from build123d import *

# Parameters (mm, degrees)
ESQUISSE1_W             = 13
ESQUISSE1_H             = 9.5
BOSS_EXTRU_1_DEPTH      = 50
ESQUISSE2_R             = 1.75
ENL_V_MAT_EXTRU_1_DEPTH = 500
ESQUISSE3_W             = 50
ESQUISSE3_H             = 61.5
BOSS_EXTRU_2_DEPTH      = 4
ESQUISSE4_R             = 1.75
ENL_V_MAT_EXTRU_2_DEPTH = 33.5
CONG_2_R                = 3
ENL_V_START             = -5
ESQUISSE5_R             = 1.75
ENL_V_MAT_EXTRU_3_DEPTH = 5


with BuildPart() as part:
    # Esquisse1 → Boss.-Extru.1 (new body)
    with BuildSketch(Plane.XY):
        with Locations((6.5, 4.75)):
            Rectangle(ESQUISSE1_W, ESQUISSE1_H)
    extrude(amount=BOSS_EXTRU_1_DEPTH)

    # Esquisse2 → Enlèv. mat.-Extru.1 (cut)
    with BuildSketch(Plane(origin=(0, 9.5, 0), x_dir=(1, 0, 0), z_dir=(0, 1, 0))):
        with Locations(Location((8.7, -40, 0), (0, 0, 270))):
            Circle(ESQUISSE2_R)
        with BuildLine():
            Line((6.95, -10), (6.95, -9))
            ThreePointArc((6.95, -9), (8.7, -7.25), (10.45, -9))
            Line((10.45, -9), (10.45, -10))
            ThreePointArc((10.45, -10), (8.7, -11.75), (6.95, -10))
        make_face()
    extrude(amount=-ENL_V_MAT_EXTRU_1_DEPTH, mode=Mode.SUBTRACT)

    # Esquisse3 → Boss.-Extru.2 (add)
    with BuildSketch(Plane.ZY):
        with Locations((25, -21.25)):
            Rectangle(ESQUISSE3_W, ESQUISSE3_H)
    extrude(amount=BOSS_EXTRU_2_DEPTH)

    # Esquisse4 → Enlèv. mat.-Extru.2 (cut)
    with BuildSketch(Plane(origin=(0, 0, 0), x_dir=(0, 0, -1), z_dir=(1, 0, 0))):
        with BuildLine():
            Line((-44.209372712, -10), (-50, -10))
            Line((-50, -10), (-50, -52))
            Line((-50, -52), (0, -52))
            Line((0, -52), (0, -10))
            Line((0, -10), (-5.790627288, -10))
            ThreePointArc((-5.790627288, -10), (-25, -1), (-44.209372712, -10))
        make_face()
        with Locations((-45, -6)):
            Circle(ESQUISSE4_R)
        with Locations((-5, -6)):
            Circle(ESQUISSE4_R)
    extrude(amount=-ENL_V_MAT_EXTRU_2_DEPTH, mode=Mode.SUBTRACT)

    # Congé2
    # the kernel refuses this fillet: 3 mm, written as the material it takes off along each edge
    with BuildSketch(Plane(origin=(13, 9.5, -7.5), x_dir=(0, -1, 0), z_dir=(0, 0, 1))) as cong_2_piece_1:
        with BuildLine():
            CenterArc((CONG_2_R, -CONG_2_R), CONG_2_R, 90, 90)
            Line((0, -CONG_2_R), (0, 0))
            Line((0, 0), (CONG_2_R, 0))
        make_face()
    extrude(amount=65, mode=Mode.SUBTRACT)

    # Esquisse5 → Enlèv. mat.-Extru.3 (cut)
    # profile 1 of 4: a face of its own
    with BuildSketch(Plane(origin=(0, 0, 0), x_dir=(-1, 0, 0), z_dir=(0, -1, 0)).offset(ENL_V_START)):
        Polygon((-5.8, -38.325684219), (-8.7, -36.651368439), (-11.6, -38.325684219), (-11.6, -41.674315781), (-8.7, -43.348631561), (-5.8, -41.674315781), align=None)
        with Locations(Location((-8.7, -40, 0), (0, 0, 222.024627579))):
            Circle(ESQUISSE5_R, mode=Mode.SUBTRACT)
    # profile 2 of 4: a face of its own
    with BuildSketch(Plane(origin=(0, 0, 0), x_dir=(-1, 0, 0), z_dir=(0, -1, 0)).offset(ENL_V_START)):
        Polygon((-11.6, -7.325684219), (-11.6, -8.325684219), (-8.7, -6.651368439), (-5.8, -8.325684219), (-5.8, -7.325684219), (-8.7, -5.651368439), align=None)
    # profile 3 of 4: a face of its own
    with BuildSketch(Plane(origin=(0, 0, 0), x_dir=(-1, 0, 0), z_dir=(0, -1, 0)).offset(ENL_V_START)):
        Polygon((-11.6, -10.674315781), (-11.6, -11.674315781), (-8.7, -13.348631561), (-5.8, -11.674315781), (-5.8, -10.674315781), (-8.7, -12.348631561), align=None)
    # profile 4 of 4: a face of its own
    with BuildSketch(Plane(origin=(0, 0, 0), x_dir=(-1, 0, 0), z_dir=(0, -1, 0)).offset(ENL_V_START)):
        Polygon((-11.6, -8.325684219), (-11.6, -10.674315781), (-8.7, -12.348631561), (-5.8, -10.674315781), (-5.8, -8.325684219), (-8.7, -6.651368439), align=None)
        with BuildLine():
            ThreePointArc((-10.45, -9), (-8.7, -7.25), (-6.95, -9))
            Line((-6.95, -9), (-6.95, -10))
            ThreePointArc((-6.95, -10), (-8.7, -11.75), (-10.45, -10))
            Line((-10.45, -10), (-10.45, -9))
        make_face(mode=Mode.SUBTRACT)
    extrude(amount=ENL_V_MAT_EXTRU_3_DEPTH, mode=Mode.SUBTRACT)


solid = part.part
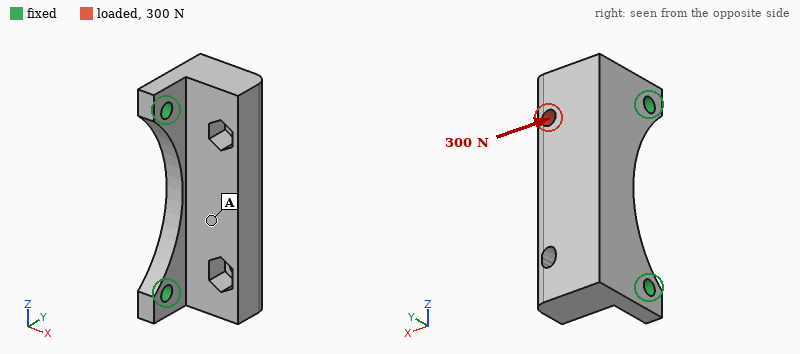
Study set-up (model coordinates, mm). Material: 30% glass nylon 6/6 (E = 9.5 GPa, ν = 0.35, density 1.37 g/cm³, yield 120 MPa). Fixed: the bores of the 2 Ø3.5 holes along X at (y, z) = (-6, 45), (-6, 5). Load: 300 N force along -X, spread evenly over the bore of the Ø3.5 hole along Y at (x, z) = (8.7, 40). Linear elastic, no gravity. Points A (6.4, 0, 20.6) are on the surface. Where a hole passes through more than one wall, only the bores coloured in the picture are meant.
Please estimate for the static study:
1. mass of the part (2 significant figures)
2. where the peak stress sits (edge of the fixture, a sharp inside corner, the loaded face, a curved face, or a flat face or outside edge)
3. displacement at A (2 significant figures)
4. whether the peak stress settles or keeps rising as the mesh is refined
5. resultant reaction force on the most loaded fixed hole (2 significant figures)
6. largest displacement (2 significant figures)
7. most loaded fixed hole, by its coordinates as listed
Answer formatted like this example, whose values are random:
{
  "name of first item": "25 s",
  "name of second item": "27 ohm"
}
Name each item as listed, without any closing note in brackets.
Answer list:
{
  "mass of the part": "12 g",
  "where the peak stress sits": "edge of the fixture",
  "displacement at A": "0.15 mm",
  "whether the peak stress settles or keeps rising as the mesh is refined": "keeps rising",
  "resultant reaction force on the most loaded fixed hole": "260 N",
  "largest displacement": "0.35 mm",
  "most loaded fixed hole, by its coordinates as listed": "(-6, 45)"
}
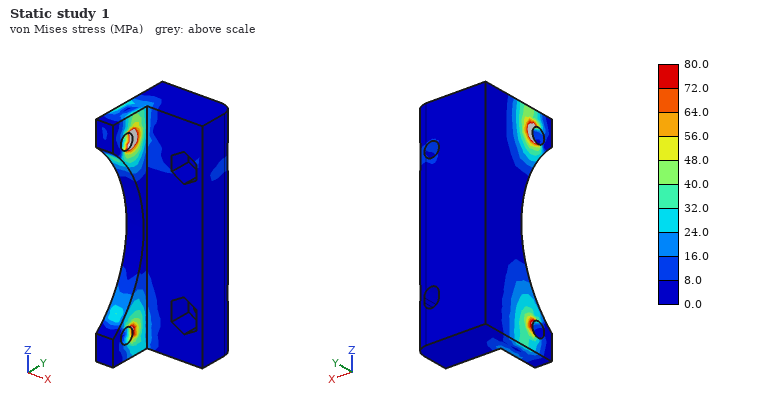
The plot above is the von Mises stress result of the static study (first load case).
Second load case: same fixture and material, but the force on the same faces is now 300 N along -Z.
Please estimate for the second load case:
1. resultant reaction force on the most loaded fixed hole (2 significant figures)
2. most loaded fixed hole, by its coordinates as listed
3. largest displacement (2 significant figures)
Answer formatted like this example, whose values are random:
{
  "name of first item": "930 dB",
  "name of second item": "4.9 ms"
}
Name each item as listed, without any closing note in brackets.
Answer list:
{
  "resultant reaction force on the most loaded fixed hole": "200 N",
  "most loaded fixed hole, by its coordinates as listed": "(-6, 5)",
  "largest displacement": "31 µm"
}
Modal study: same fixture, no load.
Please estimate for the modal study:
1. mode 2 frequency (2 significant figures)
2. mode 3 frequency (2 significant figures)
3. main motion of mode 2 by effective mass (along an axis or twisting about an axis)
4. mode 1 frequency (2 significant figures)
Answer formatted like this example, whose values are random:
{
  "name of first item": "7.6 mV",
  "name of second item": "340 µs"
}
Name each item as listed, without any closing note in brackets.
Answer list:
{
  "mode 2 frequency": "5700 Hz",
  "mode 3 frequency": "7500 Hz",
  "main motion of mode 2 by effective mass": "along Z",
  "mode 1 frequency": "1800 Hz"
}
